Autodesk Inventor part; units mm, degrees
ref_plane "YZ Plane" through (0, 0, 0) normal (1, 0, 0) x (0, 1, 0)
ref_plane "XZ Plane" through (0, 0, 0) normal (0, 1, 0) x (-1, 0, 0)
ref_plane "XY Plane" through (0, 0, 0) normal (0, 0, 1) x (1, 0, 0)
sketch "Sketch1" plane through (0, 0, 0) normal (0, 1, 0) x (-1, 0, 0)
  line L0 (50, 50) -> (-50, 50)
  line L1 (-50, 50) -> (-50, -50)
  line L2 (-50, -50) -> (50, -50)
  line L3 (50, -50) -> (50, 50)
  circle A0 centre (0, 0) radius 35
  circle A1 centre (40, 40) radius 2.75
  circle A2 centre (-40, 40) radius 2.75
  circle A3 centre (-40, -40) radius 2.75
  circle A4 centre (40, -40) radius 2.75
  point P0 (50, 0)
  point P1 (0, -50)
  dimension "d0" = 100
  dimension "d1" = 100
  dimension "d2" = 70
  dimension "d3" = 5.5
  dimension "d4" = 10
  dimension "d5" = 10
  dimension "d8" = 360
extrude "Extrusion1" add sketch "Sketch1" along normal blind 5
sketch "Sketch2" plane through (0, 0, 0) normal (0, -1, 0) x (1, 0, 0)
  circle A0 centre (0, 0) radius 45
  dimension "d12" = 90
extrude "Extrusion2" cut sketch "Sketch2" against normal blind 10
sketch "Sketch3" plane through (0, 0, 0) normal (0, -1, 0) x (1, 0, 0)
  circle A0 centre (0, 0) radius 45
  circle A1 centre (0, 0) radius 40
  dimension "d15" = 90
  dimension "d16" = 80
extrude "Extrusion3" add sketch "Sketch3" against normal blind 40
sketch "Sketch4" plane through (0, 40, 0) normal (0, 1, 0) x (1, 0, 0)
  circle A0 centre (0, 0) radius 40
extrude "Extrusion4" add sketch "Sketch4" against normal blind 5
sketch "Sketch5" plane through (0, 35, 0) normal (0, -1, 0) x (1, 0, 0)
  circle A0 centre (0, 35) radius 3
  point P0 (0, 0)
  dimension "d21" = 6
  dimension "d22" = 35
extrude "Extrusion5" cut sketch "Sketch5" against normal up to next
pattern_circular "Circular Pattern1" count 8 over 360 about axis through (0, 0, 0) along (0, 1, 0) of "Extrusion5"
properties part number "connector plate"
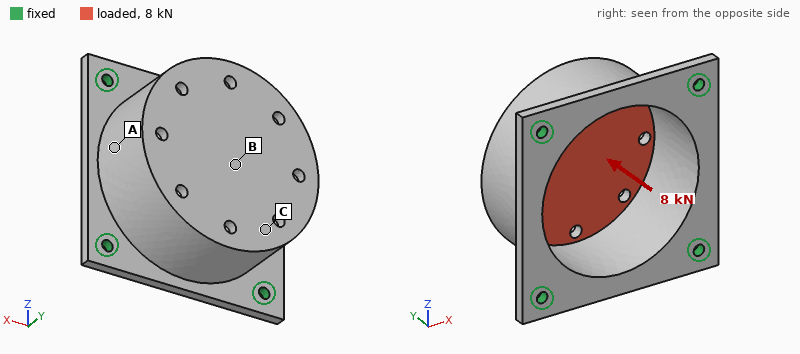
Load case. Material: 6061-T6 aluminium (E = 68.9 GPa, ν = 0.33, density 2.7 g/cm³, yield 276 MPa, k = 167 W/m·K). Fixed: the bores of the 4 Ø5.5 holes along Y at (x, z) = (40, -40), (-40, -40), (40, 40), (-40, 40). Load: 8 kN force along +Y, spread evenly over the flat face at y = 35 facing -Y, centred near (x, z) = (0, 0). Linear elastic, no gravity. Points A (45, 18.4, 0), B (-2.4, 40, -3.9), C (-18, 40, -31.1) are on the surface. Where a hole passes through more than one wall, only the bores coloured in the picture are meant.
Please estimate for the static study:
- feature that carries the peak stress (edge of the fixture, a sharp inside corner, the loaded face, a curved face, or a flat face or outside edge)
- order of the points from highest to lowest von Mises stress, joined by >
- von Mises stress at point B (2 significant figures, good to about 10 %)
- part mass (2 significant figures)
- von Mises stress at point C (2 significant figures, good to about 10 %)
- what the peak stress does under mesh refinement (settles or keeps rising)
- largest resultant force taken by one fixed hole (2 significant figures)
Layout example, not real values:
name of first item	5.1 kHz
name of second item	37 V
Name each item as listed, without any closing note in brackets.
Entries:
feature that carries the peak stress	edge of the fixture
order of the points from highest to lowest von Mises stress, joined by >	B > C > A
von Mises stress at point B	75 MPa
part mass	260 g
von Mises stress at point C	43 MPa
what the peak stress does under mesh refinement	keeps rising
largest resultant force taken by one fixed hole	2.2 kN
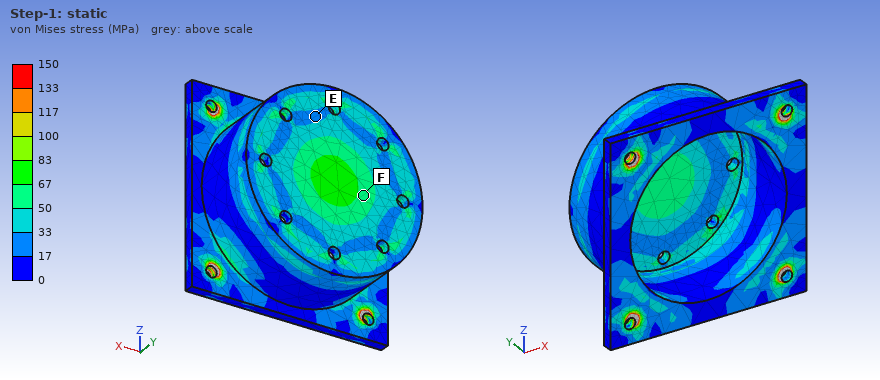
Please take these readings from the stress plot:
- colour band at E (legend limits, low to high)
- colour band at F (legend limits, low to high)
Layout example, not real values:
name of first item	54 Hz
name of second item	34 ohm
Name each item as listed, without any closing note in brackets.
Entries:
colour band at E	17 to 33 MPa
colour band at F	50 to 67 MPa
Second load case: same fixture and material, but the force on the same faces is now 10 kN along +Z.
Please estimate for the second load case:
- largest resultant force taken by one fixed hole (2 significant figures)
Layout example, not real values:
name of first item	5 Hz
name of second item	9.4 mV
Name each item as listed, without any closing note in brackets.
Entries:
largest resultant force taken by one fixed hole	3.4 kN
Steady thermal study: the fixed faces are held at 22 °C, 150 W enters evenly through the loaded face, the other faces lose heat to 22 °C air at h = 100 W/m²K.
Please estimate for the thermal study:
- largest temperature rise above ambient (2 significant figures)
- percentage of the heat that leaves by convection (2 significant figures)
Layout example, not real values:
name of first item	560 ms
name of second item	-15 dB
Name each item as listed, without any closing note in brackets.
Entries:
largest temperature rise above ambient	44 K
percentage of the heat that leaves by convection	48 %
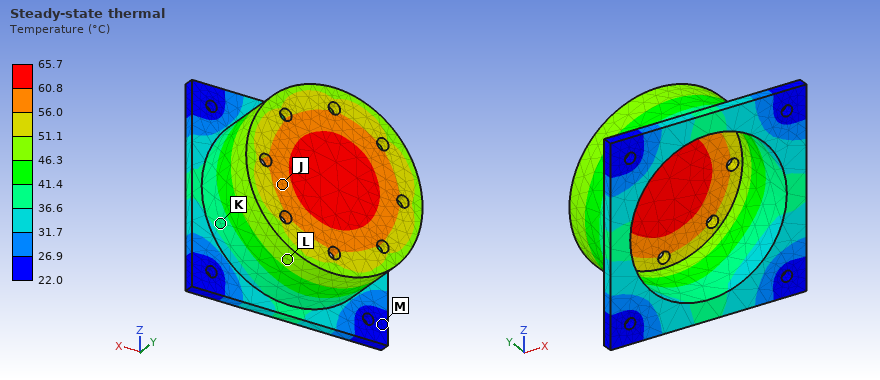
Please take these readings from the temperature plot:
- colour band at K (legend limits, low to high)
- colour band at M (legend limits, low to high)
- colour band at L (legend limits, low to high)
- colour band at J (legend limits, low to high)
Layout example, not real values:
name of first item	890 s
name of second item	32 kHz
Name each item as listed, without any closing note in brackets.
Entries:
colour band at K	36.6 to 41.4 °C
colour band at M	22.0 to 26.9 °C
colour band at L	46.3 to 51.1 °C
colour band at J	56.0 to 60.8 °C
